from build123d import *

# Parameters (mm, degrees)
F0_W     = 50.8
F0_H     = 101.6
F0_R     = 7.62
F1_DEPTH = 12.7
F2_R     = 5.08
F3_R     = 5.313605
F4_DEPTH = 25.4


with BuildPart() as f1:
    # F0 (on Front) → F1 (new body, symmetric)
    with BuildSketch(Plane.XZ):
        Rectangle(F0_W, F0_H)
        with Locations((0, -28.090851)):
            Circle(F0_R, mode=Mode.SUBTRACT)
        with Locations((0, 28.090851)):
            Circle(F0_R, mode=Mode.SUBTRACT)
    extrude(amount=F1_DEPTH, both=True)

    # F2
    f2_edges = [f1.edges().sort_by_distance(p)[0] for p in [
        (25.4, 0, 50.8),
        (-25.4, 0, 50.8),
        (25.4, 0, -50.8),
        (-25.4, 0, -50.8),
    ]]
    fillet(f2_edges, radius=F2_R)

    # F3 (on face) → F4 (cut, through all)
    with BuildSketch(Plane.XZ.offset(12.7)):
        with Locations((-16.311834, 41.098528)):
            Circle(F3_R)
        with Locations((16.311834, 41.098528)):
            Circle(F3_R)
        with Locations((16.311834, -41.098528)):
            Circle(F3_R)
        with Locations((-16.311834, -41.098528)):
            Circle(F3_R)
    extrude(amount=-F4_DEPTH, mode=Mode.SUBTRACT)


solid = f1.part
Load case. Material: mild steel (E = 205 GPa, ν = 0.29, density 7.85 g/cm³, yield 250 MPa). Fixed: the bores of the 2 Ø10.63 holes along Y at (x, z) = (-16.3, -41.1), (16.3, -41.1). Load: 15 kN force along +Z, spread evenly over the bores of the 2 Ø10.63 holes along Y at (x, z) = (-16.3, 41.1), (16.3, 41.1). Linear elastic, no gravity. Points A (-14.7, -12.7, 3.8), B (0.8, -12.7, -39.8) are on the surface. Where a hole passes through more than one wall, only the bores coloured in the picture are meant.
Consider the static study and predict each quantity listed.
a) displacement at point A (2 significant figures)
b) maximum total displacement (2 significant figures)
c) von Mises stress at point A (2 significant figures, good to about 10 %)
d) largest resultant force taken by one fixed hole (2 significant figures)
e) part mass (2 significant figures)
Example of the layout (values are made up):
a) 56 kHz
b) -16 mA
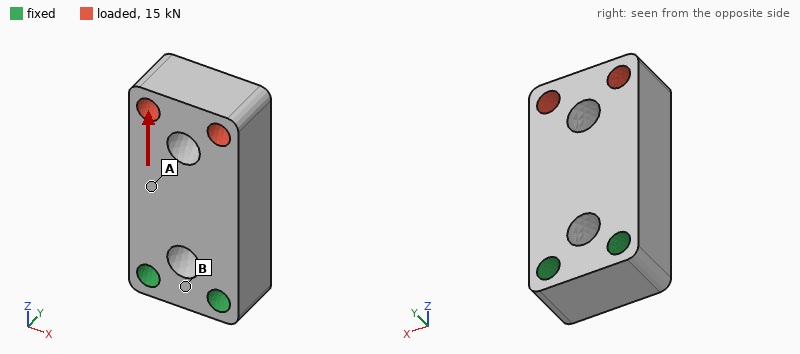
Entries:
a) 2.9 µm
b) 7.3 µm
c) 12 MPa
d) 7.5 kN
e) 880 g
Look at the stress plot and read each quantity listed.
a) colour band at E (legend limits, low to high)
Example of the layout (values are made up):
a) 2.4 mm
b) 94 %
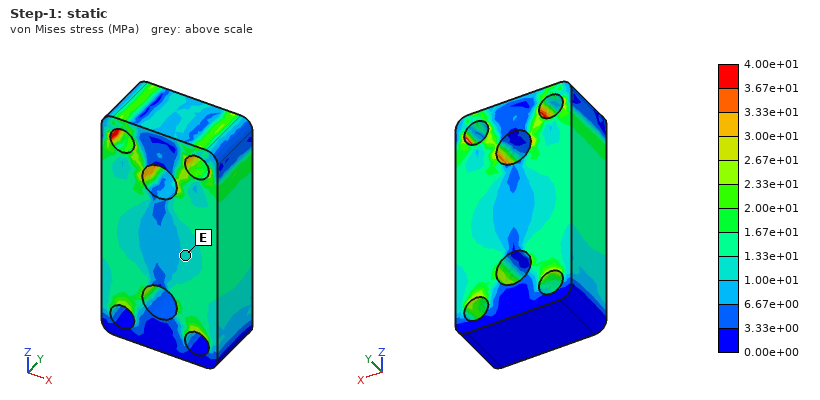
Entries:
a) 1.00e+01 to 1.33e+01 MPa
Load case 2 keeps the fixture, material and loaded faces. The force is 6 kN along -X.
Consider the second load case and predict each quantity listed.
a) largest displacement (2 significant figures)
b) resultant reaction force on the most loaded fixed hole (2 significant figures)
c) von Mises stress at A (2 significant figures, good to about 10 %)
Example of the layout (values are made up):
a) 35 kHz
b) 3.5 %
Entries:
a) 31 µm
b) 13 kN
c) 13 MPa
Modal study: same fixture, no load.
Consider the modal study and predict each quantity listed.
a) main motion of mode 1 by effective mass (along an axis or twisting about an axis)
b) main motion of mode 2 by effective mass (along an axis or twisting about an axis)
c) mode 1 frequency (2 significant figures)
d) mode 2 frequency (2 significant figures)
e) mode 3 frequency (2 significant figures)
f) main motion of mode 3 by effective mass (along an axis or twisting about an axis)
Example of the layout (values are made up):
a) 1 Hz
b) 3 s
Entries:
a) along Y
b) along X
c) 2500 Hz
d) 4500 Hz
e) 7000 Hz
f) twisting about Z
